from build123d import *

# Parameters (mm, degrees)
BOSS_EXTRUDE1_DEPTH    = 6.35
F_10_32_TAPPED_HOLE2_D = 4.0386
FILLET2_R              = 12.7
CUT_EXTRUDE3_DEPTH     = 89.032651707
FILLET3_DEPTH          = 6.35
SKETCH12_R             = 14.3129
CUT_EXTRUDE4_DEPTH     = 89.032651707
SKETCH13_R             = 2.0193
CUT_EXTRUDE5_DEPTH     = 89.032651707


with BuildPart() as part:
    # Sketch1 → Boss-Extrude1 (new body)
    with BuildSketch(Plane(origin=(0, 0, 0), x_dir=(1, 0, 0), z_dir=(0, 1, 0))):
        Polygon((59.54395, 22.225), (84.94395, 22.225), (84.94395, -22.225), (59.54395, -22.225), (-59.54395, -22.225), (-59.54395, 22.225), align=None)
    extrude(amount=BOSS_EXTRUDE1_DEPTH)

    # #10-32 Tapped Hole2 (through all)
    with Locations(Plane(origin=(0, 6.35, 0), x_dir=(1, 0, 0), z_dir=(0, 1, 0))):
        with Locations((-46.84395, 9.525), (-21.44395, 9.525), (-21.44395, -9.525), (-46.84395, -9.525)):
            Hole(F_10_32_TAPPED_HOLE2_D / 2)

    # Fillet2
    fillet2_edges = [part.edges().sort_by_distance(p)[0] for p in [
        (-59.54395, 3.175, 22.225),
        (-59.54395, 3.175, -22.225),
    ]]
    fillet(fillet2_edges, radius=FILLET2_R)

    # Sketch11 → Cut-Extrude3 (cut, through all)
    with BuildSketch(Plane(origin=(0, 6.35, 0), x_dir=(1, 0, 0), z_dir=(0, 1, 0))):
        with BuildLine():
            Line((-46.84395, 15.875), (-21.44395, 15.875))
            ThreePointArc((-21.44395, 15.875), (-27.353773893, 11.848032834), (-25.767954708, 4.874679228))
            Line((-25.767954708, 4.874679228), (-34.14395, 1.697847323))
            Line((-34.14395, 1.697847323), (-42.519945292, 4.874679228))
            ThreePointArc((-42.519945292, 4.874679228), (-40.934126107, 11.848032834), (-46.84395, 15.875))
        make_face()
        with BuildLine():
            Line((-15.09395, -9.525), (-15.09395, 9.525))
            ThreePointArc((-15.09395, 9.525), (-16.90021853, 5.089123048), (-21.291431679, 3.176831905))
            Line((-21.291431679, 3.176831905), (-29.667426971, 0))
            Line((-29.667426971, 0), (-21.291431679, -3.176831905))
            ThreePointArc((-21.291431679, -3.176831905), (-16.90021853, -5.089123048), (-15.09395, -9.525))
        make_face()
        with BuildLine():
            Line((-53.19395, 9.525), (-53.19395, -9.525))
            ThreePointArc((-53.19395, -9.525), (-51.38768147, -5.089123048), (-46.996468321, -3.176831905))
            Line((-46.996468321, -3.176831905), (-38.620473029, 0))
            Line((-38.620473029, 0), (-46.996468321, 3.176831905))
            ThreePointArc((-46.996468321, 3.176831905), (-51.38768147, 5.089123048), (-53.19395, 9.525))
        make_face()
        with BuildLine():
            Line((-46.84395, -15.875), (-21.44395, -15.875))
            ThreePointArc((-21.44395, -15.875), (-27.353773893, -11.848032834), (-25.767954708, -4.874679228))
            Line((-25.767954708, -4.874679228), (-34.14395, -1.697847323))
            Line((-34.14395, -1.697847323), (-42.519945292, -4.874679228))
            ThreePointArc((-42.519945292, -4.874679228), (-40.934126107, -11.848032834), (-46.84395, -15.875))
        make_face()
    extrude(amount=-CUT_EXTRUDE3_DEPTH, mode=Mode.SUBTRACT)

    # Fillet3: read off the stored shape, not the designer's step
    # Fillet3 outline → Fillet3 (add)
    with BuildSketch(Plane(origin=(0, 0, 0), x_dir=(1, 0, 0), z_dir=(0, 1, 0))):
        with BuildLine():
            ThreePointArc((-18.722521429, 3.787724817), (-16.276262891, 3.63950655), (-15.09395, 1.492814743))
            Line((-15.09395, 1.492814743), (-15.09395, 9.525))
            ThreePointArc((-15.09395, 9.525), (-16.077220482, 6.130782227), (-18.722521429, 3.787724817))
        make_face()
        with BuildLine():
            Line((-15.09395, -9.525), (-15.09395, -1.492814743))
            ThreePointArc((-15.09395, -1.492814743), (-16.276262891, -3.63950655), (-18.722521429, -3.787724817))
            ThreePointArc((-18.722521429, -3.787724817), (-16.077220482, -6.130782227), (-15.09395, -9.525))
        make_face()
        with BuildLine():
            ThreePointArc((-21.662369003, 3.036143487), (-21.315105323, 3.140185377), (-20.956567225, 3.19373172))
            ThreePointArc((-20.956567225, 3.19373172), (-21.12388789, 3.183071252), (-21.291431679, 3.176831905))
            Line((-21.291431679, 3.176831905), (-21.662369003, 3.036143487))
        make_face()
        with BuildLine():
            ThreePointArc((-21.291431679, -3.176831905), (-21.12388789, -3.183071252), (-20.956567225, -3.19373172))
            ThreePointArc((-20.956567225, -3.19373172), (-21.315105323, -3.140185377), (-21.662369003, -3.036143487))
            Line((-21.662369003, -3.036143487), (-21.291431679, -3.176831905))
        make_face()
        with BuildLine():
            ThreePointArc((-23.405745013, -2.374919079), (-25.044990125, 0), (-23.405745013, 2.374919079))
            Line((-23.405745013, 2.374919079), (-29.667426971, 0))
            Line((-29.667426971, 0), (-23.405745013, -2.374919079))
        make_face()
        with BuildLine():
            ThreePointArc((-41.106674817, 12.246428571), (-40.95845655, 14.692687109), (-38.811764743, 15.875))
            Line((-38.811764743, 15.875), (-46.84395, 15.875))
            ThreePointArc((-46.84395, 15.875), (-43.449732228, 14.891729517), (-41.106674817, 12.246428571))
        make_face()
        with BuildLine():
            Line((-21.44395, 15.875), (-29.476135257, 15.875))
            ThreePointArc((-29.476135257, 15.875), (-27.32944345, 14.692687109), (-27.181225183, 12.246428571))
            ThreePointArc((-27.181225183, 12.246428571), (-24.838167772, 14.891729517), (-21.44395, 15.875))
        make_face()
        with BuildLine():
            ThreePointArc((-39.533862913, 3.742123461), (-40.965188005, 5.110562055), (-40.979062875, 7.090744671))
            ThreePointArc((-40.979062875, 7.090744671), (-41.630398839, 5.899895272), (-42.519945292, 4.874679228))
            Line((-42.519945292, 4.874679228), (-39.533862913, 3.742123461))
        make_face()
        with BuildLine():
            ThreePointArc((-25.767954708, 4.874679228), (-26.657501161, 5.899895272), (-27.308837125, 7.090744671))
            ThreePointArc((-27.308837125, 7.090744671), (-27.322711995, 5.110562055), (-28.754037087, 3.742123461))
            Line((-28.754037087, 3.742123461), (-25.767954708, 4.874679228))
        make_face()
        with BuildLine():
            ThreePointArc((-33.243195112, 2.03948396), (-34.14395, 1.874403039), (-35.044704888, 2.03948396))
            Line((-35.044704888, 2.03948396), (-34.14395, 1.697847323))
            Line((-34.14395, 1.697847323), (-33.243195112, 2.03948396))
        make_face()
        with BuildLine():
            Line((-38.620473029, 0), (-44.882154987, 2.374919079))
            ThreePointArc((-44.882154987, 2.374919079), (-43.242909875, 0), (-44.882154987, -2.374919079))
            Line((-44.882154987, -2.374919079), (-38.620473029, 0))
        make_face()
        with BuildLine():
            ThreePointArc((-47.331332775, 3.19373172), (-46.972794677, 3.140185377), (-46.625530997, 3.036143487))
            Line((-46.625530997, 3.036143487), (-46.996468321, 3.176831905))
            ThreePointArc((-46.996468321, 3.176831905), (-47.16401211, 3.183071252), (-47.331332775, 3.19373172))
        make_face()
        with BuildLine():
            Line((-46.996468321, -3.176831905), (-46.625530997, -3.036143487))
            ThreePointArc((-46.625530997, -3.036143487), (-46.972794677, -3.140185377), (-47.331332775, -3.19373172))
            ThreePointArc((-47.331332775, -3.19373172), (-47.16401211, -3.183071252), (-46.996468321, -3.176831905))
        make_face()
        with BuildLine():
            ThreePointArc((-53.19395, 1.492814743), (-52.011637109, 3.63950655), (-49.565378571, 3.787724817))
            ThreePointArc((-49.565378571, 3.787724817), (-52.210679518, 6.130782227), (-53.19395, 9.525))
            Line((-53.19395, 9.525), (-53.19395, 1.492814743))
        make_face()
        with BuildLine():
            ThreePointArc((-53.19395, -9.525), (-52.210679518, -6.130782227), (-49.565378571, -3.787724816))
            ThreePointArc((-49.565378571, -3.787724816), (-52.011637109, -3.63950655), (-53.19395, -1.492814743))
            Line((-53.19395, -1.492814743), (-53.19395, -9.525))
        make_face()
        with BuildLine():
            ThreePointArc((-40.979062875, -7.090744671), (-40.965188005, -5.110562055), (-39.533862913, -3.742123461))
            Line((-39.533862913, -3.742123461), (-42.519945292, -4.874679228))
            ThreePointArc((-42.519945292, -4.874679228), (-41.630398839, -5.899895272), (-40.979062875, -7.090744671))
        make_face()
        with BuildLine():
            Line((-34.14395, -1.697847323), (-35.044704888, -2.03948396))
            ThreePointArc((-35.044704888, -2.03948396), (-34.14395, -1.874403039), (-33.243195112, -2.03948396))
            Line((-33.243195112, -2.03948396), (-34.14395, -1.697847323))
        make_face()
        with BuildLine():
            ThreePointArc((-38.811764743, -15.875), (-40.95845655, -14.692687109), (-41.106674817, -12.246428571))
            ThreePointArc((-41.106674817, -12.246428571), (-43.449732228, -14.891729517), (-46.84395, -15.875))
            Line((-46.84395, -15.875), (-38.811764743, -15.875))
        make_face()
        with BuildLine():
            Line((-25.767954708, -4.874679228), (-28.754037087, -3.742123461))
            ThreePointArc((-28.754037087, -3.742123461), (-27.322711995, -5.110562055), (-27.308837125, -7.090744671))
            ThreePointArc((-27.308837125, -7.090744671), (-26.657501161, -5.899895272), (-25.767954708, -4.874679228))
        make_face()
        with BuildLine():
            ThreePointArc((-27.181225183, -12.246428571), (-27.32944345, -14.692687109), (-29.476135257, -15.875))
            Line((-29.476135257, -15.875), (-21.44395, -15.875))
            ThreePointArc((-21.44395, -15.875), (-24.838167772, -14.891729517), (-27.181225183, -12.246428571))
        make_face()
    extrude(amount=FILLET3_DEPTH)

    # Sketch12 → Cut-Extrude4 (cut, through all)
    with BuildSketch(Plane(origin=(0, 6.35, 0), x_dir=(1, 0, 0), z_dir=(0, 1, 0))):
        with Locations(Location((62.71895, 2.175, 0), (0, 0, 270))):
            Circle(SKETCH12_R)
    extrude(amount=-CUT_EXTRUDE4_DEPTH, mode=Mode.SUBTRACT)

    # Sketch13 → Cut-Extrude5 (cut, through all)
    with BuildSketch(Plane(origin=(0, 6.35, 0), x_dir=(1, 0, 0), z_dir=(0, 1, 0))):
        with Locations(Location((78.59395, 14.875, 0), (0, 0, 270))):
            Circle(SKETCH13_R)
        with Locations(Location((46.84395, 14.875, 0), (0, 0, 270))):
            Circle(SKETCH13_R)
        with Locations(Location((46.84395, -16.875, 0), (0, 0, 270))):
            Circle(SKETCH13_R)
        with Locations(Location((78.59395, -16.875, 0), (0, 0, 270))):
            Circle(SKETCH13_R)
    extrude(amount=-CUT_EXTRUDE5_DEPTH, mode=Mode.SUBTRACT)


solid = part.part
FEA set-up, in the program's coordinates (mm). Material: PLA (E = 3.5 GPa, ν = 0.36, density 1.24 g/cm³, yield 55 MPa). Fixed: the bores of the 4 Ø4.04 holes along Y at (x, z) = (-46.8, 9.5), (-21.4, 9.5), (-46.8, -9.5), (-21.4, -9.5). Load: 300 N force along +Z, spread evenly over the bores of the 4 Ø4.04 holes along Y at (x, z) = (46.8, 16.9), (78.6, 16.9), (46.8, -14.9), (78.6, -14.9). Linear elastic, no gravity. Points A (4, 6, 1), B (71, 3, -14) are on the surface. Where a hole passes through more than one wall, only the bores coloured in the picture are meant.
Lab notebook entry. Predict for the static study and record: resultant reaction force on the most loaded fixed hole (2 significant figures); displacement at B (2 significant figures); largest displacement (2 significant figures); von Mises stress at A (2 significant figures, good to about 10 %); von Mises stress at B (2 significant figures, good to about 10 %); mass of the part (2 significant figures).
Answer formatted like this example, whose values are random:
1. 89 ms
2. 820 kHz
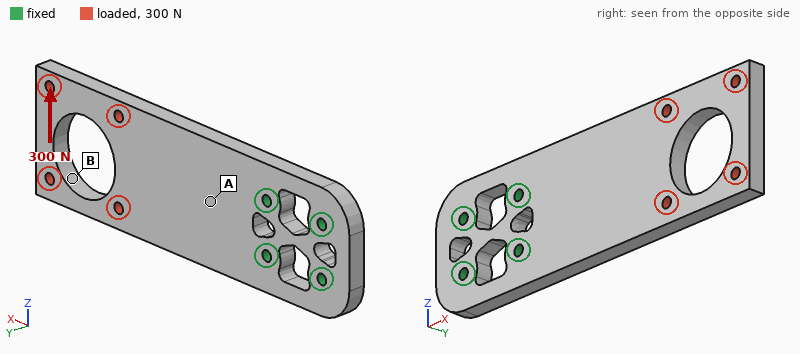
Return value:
1. 810 N
2. 0.82 mm
3. 0.98 mm
4. 3.4 MPa
5. 9.3 MPa
6. 40 g
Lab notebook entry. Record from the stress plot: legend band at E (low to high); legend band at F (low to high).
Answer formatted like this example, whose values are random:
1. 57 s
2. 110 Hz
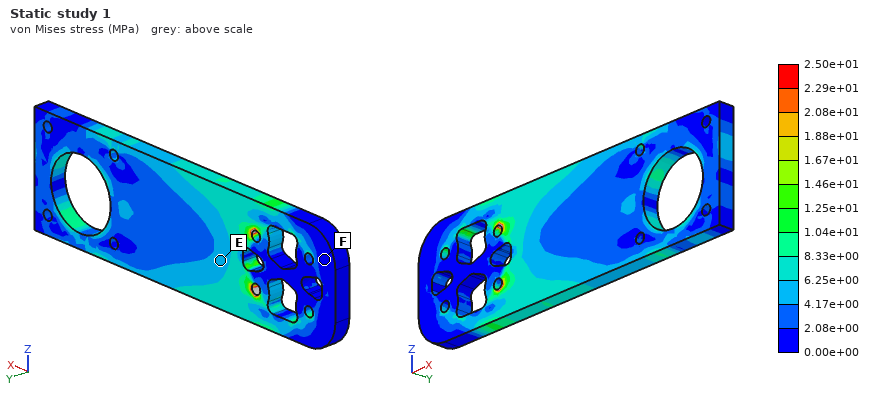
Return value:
1. 4.17e+00 to 6.25e+00 MPa
2. 0.00e+00 to 2.08e+00 MPa
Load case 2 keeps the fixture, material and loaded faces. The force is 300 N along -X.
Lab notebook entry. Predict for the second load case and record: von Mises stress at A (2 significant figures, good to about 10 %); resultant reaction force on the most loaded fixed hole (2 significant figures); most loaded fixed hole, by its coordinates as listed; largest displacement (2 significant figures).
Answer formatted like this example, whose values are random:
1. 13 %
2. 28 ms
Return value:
1. 1.1 MPa
2. 140 N
3. (-21.4, 9.5)
4. 52 µm
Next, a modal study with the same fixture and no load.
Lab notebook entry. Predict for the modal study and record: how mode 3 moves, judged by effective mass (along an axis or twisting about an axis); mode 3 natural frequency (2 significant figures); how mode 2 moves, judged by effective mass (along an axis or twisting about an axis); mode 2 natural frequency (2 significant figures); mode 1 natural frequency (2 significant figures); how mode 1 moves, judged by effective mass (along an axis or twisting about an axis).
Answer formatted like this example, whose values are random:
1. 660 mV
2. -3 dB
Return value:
1. along Y
2. 840 Hz
3. twisting about X
4. 700 Hz
5. 180 Hz
6. along Y
